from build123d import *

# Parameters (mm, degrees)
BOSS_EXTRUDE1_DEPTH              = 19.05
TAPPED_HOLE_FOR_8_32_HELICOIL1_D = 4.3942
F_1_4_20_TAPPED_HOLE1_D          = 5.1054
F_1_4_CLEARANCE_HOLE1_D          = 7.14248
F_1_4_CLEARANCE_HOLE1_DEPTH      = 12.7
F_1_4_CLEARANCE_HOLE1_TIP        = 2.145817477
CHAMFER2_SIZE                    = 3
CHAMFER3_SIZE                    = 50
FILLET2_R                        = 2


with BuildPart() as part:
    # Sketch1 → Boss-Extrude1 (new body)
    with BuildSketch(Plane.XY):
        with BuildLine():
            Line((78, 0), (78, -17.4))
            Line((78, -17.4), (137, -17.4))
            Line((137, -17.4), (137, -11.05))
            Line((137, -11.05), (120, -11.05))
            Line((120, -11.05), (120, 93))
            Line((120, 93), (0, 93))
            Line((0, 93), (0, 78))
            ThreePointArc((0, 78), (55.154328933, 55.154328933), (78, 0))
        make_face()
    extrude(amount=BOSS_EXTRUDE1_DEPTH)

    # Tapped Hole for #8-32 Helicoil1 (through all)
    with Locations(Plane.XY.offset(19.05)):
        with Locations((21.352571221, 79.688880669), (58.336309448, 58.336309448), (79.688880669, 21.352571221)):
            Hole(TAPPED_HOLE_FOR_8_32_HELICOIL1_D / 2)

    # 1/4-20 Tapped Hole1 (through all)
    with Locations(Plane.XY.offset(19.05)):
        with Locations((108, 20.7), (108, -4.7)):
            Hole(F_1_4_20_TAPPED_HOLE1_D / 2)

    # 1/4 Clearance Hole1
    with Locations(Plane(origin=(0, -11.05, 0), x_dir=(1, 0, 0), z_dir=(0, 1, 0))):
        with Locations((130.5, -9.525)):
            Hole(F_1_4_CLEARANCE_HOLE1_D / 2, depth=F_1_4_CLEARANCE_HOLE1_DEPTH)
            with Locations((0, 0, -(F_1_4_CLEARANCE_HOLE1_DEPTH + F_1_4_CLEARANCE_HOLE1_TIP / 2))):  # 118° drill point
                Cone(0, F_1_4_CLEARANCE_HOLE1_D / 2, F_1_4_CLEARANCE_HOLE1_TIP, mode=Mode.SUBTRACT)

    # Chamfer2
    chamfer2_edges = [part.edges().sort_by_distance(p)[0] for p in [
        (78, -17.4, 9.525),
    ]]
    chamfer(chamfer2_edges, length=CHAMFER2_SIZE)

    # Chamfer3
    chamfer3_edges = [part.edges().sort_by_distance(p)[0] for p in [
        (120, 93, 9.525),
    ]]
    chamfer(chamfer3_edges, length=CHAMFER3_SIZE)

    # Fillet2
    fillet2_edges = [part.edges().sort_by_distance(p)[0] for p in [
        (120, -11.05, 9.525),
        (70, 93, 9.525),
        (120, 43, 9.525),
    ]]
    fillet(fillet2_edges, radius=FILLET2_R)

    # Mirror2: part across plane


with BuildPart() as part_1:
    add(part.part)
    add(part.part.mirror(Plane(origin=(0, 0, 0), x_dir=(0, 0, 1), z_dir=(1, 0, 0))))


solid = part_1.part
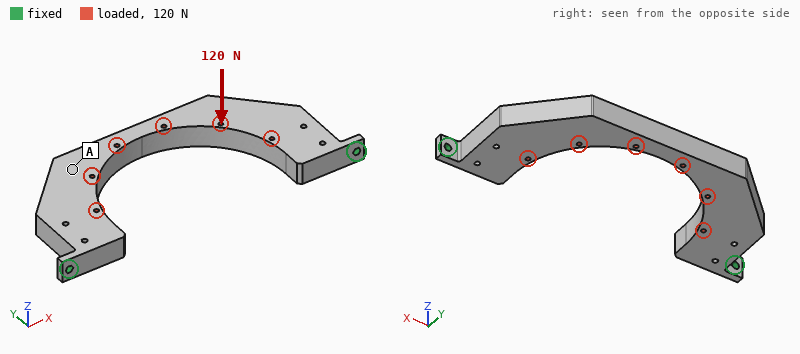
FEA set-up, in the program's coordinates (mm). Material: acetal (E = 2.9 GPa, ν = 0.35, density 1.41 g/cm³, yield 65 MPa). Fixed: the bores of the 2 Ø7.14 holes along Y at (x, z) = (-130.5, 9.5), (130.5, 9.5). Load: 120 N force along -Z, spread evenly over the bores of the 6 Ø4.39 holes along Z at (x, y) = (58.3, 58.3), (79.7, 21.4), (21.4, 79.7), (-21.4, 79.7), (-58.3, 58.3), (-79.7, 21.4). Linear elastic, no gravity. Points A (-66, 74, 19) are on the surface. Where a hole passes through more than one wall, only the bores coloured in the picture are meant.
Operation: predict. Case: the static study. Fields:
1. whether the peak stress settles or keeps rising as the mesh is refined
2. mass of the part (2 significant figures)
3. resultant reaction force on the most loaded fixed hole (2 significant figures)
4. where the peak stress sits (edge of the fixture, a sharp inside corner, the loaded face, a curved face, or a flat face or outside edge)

keeps rising
320 g
60 N
edge of the fixture
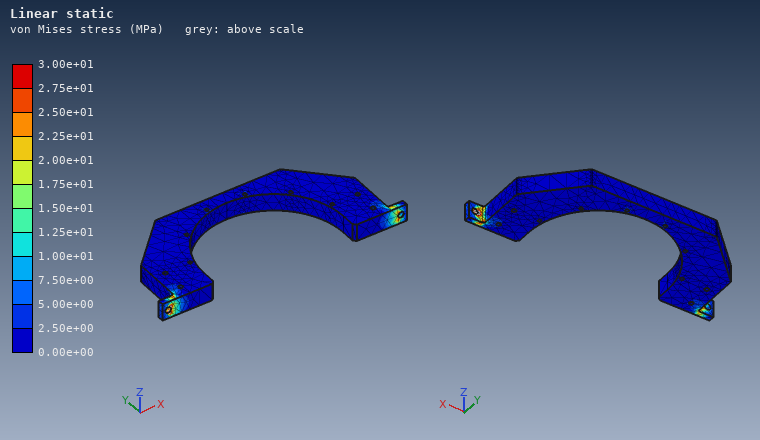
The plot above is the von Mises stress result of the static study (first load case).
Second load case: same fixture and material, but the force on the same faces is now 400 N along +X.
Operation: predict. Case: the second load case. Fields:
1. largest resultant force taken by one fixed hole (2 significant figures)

230 N
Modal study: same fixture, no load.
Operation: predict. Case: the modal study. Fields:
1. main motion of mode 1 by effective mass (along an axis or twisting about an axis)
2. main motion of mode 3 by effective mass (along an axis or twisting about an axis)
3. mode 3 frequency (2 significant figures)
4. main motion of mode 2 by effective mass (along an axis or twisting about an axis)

along Z
along X
450 Hz
twisting about Y
